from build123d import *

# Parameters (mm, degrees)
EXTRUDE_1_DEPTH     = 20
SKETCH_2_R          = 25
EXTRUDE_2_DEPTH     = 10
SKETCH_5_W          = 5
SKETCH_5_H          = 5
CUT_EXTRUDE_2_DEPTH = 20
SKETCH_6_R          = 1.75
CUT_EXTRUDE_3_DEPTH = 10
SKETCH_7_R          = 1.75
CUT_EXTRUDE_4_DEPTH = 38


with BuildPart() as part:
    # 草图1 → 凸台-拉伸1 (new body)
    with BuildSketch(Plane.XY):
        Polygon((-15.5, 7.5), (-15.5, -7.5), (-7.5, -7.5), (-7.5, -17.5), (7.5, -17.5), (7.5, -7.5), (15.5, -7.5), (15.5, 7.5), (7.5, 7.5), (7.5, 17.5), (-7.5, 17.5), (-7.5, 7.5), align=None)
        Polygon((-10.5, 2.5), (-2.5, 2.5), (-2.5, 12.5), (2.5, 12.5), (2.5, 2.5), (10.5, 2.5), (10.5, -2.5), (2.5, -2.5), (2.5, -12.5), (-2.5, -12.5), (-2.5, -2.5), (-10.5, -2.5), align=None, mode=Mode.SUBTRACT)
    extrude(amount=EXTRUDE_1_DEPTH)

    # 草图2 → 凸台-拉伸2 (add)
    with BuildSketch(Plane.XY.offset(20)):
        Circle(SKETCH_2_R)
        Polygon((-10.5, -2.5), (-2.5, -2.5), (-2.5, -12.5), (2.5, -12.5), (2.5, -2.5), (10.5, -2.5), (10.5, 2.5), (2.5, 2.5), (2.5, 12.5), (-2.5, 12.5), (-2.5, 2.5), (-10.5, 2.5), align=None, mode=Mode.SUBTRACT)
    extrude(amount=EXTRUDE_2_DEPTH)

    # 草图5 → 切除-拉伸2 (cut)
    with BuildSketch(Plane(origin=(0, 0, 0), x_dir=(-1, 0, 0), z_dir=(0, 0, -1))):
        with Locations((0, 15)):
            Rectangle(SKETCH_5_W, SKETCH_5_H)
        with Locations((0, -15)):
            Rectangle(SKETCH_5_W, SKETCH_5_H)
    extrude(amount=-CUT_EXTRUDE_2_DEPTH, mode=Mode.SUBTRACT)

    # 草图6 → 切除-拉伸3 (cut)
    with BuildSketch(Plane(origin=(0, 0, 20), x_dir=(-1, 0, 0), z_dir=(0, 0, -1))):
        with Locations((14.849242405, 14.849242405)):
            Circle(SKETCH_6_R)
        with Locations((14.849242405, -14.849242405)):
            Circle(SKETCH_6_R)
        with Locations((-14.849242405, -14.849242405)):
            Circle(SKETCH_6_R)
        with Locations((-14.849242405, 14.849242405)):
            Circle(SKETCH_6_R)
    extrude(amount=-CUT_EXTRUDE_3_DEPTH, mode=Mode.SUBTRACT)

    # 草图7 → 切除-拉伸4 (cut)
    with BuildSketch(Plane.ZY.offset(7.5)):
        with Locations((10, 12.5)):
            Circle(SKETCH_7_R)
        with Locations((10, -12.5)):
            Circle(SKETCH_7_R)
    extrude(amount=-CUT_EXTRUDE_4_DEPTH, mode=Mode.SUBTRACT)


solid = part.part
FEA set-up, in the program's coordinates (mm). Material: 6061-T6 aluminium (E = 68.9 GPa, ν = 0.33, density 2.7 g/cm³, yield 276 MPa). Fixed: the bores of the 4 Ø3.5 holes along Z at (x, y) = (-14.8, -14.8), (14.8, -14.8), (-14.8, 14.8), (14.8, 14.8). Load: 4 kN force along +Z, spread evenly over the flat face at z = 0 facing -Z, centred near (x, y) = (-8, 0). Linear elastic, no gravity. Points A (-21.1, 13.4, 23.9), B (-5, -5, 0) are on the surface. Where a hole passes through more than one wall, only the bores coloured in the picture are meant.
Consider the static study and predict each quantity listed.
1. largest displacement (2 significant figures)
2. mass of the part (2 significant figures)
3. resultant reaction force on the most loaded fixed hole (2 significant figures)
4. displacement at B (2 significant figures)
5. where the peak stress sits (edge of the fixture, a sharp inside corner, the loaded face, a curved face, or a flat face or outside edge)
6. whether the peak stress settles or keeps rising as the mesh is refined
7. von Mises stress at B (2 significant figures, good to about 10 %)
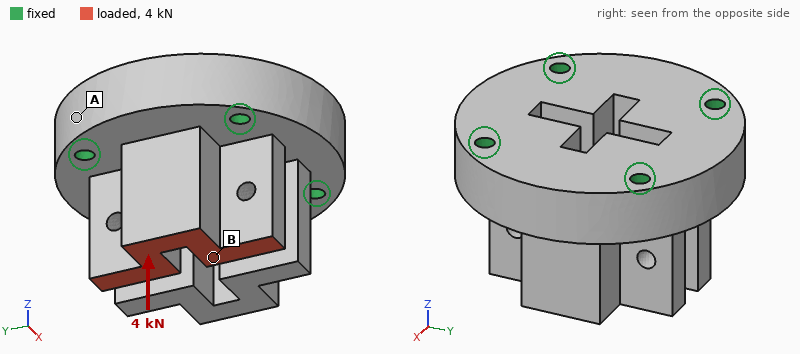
19 µm
73 g
1.6 kN
16 µm
edge of the fixture
keeps rising
15 MPa
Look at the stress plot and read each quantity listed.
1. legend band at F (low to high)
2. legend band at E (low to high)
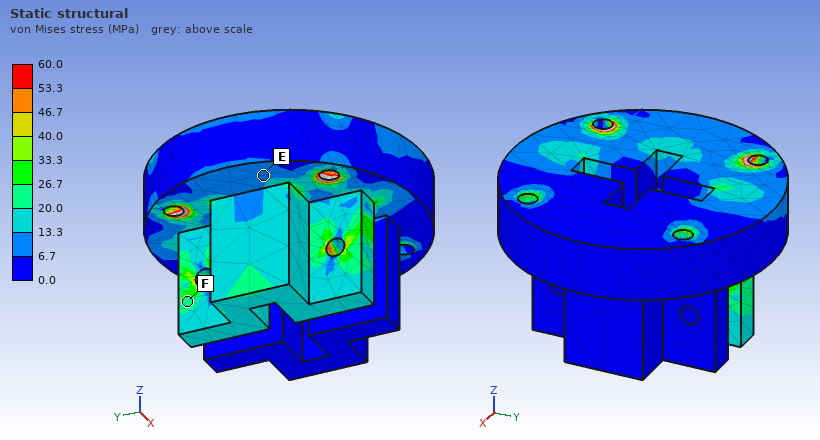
20.0 to 26.7 MPa
6.7 to 13.3 MPa
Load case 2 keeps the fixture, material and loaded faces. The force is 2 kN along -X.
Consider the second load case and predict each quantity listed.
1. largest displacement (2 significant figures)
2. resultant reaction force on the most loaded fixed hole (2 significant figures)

0.11 mm
1.1 kN
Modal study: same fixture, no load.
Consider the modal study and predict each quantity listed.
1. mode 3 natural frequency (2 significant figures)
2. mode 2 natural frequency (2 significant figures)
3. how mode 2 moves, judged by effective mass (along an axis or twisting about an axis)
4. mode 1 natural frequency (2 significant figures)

14 kHz
12 kHz
along X
10 kHz
